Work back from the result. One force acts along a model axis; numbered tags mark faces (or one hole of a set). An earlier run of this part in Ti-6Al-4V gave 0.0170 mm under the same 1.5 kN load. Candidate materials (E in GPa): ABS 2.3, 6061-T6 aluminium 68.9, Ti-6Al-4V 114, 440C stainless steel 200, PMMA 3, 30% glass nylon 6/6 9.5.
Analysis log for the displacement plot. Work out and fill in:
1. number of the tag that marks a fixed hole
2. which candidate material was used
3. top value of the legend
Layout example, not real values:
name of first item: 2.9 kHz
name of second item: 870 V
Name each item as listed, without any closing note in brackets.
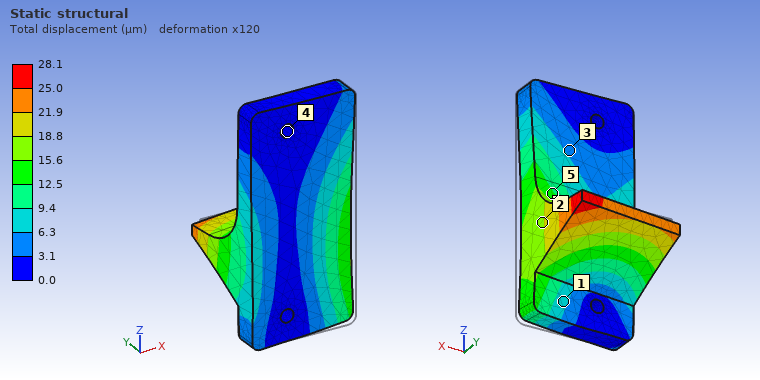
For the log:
number of the tag that marks a fixed hole: 4
which candidate material was used: 6061-T6 aluminium
top value of the legend: 28.1 µm
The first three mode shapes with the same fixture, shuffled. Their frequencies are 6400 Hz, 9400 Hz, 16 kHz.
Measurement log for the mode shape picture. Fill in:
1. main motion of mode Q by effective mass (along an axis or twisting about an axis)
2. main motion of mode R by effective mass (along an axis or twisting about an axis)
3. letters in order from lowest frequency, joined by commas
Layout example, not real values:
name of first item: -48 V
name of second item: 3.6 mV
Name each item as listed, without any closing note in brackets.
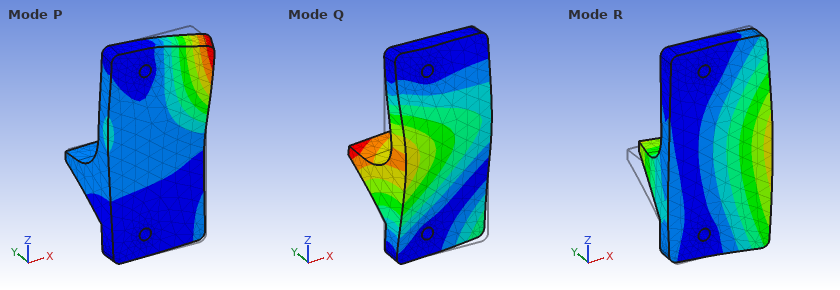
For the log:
main motion of mode Q by effective mass: along Y
main motion of mode R by effective mass: along Y
letters in order from lowest frequency, joined by commas: R, Q, P
